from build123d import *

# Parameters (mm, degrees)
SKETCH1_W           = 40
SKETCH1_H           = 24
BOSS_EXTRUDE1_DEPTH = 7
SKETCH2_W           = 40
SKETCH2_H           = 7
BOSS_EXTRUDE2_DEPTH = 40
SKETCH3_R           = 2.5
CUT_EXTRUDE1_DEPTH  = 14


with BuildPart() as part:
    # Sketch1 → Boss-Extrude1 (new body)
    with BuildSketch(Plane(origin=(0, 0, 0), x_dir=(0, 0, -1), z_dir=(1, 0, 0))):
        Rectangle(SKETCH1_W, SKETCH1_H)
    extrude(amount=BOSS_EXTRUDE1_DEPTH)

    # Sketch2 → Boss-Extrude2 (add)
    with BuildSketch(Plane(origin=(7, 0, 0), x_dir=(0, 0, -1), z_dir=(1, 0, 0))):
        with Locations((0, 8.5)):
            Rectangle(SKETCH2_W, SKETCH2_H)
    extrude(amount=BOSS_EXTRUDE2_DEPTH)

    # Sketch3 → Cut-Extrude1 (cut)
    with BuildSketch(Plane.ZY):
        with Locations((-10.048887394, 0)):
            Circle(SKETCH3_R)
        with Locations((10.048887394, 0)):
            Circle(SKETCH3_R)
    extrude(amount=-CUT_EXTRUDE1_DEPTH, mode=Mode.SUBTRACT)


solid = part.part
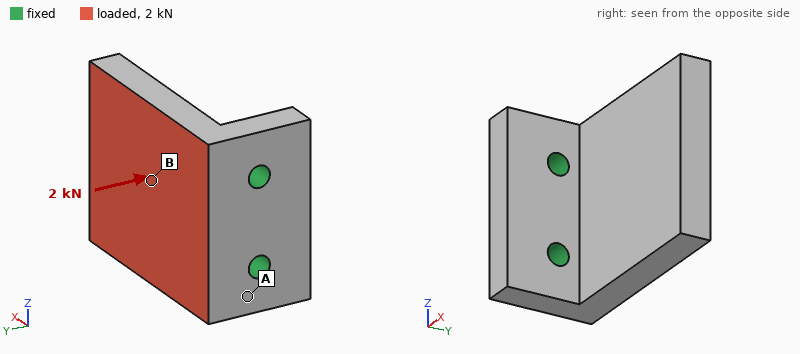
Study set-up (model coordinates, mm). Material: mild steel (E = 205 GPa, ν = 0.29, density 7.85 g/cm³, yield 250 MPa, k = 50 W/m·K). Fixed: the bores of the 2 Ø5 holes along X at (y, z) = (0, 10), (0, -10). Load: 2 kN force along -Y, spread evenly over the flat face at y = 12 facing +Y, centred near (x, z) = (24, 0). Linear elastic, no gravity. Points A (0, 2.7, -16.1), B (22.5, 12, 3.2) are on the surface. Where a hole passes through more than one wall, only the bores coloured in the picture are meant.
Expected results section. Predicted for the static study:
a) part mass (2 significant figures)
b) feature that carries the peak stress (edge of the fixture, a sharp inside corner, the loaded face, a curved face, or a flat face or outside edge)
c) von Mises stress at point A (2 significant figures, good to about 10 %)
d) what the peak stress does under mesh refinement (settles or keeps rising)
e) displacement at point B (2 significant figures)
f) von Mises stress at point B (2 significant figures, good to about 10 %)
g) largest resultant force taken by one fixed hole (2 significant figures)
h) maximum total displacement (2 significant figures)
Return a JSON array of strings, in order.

["140 g", "edge of the fixture", "77 MPa", "keeps rising", "0.047 mm", "36 MPa", "1.0 kN", "0.13 mm"]
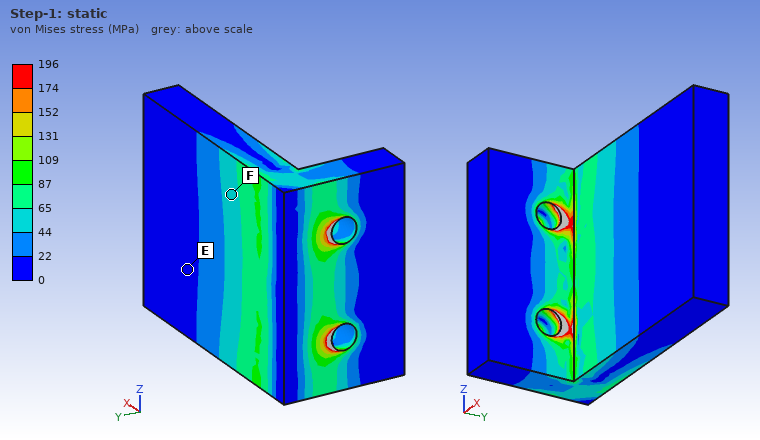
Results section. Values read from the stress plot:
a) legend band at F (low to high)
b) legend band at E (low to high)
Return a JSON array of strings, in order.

["44 to 65 MPa", "0 to 22 MPa"]
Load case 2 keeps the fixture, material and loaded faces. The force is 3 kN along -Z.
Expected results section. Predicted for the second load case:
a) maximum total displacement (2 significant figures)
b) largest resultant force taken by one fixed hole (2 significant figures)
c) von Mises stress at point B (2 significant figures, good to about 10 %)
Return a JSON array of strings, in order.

["23 µm", "3.1 kN", "24 MPa"]
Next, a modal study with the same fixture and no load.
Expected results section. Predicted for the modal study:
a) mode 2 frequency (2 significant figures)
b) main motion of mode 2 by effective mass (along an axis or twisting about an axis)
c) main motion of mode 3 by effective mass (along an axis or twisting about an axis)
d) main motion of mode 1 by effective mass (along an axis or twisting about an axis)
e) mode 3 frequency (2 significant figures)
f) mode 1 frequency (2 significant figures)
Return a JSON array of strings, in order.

["6000 Hz", "along Z", "along Z", "along Y", "7600 Hz", "2400 Hz"]
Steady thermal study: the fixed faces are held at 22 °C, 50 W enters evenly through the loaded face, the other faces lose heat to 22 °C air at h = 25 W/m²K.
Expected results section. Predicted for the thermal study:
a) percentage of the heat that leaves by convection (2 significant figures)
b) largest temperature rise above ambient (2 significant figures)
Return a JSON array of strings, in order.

["9.1 %", "84 K"]
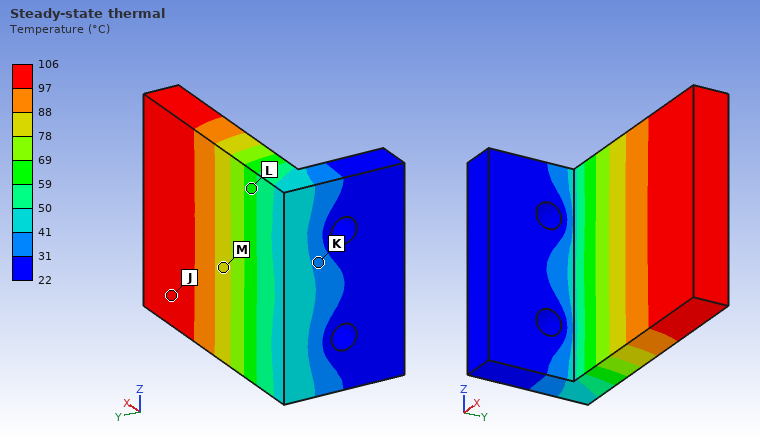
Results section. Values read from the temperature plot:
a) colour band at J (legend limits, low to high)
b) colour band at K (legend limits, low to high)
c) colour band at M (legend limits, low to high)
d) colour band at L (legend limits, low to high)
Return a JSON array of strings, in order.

["97 to 106 °C", "31 to 41 °C", "78 to 88 °C", "59 to 69 °C"]
